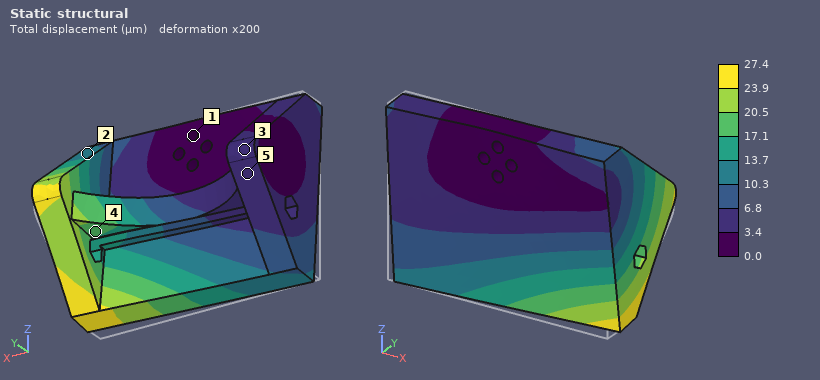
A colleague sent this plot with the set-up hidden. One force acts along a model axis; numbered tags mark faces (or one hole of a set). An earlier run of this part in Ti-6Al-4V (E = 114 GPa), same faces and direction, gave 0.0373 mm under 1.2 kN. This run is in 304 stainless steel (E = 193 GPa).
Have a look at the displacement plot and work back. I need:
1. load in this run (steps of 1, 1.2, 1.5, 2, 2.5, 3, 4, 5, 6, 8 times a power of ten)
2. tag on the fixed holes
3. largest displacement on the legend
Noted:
1.5 kN
1
27.4 µm
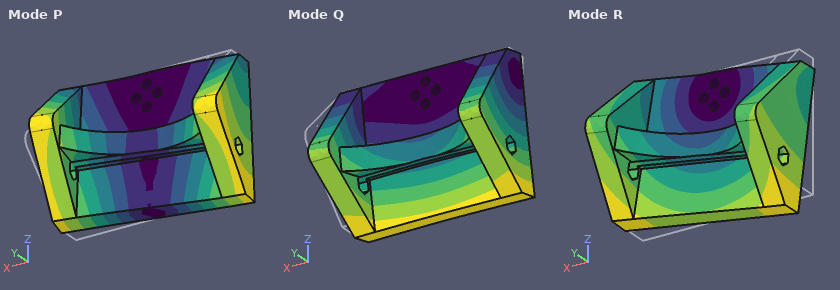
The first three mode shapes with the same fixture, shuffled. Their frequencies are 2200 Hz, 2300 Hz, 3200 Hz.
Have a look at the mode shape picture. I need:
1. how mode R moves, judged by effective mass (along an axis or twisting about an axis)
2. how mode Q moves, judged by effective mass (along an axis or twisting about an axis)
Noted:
along X
along Y
